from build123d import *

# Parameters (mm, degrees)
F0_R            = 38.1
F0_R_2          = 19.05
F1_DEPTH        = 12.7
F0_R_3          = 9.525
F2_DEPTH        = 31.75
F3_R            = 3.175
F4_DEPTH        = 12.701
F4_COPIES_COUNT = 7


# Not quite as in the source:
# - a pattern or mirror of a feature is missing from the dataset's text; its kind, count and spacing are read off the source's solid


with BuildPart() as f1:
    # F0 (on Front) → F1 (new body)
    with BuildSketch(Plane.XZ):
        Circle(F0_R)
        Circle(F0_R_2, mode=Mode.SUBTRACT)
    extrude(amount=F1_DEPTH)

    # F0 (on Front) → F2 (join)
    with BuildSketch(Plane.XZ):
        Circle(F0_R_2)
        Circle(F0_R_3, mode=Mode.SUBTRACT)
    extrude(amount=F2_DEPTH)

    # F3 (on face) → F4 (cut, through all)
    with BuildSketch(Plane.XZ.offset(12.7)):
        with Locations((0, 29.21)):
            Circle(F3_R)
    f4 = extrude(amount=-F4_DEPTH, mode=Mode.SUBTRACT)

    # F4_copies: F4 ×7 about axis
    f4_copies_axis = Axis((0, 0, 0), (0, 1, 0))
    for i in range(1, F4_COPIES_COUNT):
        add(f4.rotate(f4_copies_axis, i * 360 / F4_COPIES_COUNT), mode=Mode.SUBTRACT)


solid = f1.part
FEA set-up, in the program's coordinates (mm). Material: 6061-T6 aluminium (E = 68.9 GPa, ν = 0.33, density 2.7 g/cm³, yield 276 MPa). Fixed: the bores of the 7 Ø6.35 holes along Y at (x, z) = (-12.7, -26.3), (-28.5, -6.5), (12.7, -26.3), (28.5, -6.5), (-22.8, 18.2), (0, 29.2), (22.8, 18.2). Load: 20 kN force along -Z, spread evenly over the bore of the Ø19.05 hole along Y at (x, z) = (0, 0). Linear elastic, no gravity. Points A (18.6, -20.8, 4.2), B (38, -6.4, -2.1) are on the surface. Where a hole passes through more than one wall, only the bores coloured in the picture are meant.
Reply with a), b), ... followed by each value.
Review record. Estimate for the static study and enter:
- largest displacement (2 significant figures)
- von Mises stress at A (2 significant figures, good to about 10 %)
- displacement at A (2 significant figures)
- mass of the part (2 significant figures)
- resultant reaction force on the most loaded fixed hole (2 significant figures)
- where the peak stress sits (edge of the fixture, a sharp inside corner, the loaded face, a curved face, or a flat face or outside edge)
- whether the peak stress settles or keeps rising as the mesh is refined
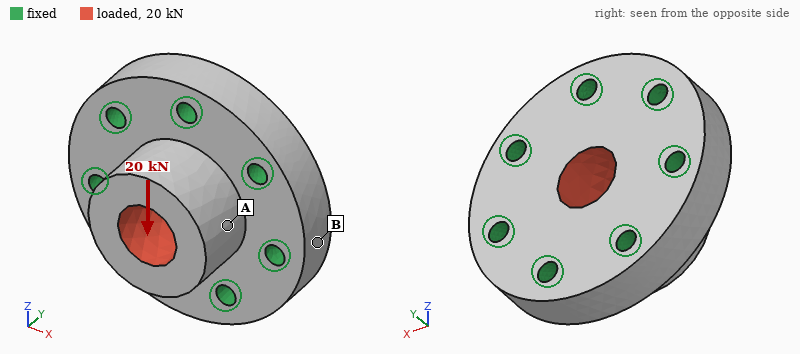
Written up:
a) 22 µm
b) 15 MPa
c) 11 µm
d) 180 g
e) 4.9 kN
f) edge of the fixture
g) keeps rising
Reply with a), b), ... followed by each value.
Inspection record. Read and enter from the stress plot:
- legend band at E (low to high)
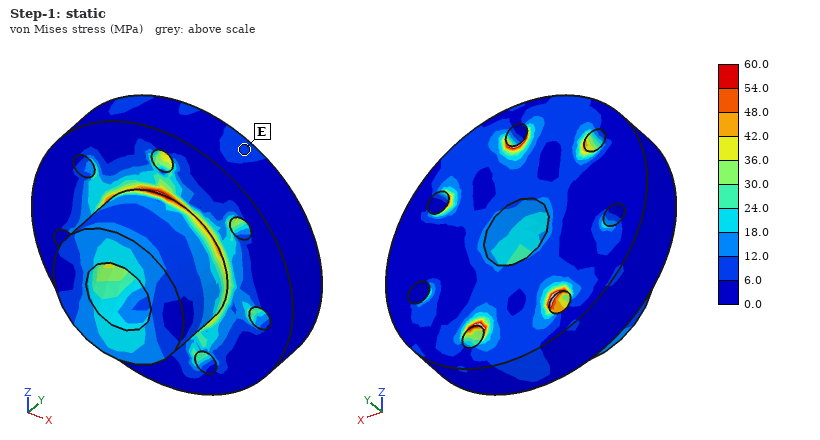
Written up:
a) 6.0 to 12.0 MPa
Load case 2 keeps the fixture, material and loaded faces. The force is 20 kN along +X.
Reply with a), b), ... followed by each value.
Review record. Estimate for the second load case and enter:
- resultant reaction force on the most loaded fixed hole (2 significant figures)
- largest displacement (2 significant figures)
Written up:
a) 4.8 kN
b) 22 µm
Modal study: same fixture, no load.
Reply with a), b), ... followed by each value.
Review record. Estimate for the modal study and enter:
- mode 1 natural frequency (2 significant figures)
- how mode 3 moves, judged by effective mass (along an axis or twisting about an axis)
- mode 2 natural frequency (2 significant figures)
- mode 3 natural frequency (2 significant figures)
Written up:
a) 21 kHz
b) along Y
c) 21 kHz
d) 23 kHz
